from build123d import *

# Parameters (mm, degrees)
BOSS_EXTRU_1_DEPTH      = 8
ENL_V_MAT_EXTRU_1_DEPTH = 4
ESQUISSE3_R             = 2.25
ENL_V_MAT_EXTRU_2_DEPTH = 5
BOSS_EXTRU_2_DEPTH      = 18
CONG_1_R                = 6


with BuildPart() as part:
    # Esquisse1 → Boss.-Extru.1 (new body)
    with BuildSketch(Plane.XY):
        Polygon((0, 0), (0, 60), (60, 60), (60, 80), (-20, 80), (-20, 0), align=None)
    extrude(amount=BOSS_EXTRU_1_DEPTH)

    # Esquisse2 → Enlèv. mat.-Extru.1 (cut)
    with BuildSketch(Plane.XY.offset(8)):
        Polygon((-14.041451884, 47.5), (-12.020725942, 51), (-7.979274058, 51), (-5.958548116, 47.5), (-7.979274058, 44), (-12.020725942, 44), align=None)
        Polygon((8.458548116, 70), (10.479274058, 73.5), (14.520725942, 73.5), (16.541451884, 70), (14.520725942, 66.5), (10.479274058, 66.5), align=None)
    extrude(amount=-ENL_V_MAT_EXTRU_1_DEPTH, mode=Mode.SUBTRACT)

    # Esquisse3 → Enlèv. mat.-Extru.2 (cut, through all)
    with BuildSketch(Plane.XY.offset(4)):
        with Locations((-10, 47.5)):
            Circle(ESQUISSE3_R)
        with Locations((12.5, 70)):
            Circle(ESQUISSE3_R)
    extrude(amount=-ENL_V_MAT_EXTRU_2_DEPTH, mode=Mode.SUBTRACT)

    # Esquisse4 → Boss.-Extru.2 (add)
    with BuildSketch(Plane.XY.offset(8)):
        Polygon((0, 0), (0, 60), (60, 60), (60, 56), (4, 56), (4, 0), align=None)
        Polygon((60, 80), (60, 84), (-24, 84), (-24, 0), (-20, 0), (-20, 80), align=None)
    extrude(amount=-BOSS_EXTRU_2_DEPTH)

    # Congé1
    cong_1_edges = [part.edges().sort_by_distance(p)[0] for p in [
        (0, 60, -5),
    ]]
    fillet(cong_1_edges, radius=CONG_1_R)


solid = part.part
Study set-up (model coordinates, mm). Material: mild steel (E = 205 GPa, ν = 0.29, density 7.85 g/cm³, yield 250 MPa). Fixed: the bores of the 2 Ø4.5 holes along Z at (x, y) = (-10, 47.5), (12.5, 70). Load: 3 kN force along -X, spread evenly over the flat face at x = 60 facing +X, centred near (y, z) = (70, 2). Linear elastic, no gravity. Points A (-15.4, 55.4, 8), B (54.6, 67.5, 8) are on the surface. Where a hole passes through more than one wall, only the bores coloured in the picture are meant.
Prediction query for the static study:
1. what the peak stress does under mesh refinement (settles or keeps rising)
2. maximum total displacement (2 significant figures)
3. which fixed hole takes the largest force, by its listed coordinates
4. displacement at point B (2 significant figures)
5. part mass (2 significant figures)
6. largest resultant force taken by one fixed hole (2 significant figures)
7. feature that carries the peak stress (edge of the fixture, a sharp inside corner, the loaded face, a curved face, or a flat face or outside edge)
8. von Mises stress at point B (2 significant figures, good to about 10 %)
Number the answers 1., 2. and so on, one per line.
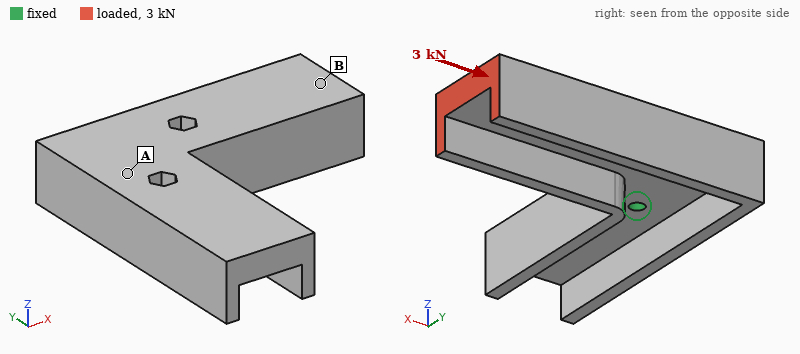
1. keeps rising
2. 5.2 µm
3. (12.5, 70)
4. 3.5 µm
5. 330 g
6. 2.7 kN
7. edge of the fixture
8. 10.0 MPa
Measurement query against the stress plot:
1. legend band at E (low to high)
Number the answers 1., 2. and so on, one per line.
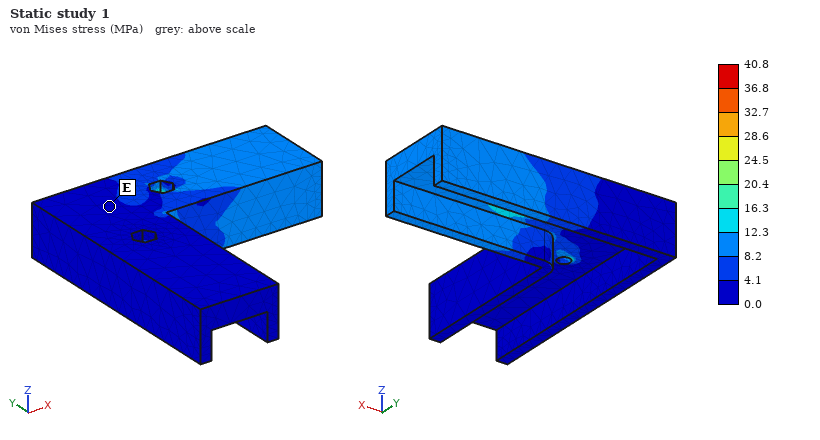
1. 0.0 to 4.1 MPa
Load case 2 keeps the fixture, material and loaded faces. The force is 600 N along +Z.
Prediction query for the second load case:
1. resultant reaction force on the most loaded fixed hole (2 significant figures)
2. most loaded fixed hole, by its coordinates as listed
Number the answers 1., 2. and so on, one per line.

1. 1.2 kN
2. (12.5, 70)
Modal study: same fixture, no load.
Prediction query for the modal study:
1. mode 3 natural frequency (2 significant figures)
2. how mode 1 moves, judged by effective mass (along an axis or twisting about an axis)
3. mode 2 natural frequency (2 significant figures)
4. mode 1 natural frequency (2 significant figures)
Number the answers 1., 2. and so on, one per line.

1. 4800 Hz
2. along Z
3. 3300 Hz
4. 2000 Hz
